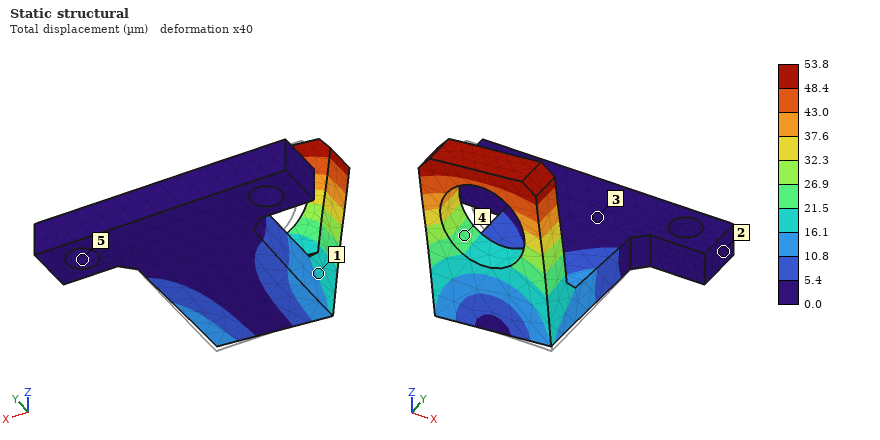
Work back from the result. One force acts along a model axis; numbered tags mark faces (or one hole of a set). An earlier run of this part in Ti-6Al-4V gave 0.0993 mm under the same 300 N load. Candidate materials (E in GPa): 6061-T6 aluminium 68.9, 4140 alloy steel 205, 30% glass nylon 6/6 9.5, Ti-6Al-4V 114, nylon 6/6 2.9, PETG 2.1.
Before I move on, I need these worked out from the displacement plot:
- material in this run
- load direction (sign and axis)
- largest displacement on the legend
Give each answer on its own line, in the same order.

4140 alloy steel
-X
53.8 µm
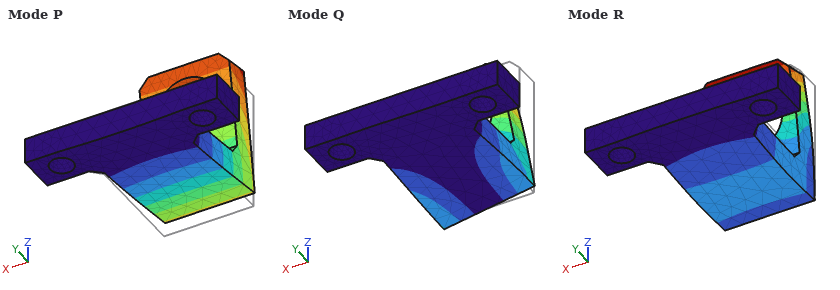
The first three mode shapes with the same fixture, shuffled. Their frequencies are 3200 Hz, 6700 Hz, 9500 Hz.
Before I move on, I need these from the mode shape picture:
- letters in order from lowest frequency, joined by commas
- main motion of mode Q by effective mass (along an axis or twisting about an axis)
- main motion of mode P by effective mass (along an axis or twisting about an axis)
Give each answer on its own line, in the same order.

P, Q, R
along X
along Z
